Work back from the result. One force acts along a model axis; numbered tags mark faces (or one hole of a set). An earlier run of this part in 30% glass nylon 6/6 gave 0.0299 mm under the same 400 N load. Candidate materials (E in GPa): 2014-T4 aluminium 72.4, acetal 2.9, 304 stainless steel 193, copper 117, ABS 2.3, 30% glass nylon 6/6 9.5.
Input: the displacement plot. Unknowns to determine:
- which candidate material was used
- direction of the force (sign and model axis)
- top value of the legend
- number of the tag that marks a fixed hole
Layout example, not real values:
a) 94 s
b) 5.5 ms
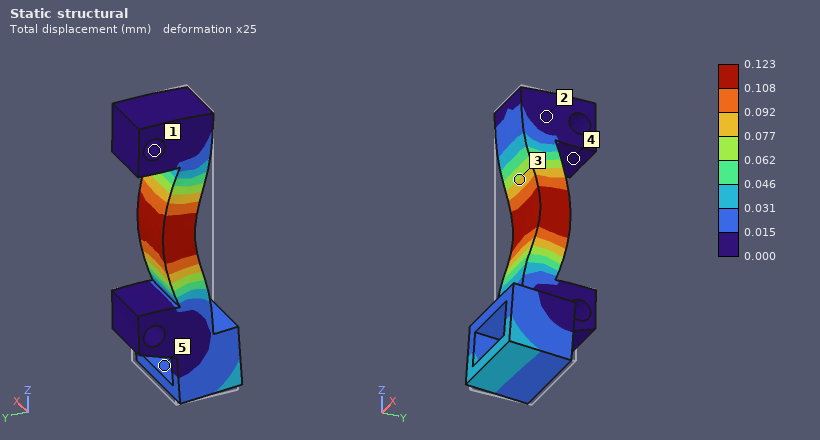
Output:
a) ABS
b) +Y
c) 0.123 mm
d) 1
